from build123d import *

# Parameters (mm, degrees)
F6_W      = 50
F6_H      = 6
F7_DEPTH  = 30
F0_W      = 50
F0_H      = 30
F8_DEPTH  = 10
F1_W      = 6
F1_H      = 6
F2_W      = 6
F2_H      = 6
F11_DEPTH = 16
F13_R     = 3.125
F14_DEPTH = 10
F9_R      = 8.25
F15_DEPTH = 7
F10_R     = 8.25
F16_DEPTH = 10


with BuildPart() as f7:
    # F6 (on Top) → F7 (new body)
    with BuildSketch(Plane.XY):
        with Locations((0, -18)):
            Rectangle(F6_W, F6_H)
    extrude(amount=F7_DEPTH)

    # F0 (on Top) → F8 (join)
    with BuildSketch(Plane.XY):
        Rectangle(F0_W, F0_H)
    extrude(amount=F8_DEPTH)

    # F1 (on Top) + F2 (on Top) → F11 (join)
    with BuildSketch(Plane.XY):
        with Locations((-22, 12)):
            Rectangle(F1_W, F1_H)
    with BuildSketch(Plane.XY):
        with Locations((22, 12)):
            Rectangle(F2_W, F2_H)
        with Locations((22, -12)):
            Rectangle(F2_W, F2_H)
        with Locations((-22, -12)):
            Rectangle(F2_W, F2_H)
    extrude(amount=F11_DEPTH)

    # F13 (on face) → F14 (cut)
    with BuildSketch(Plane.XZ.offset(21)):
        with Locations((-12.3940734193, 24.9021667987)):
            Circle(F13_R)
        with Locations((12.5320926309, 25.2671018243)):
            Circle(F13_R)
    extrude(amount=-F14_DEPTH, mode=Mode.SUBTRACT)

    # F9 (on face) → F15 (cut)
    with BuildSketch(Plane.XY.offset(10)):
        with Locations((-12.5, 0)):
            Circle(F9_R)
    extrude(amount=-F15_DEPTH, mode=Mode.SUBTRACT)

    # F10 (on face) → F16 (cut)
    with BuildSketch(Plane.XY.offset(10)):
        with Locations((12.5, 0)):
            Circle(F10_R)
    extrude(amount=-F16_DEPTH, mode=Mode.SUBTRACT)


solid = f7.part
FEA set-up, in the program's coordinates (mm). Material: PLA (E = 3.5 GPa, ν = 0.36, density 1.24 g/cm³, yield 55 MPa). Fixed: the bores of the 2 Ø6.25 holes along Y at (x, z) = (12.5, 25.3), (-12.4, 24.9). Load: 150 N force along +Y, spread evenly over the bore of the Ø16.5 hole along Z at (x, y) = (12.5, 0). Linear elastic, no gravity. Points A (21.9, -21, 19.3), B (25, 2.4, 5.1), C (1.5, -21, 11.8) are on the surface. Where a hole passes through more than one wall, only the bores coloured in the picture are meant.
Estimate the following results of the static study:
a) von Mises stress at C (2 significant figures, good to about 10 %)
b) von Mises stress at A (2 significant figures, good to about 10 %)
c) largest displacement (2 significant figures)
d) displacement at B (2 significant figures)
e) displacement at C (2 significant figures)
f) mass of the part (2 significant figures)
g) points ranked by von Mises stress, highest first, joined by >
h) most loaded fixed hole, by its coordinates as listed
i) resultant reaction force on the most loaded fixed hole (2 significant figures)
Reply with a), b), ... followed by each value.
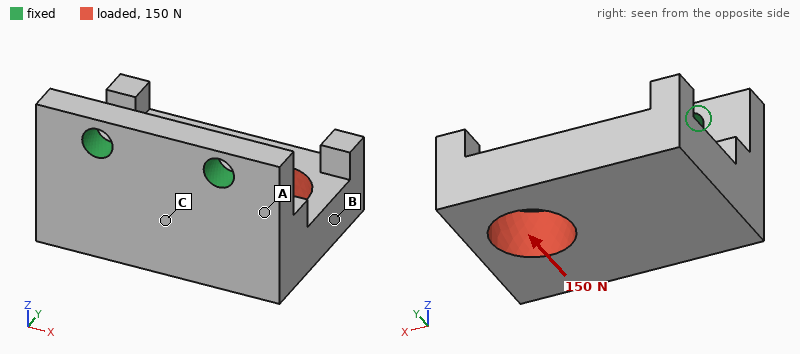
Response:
a) 3.2 MPa
b) 5.8 MPa
c) 0.38 mm
d) 0.27 mm
e) 0.072 mm
f) 26 g
g) A > C > B
h) (12.5, 25.3)
i) 130 N
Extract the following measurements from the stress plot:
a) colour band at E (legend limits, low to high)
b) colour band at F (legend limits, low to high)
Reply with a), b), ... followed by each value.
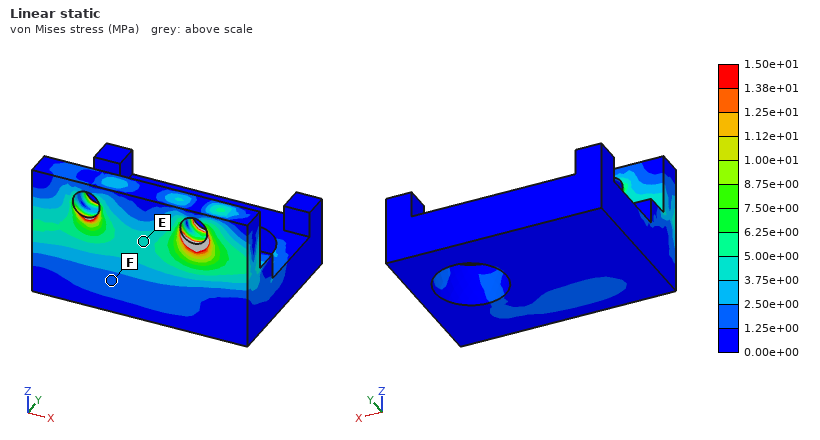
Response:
a) 3.75e+00 to 5.00e+00 MPa
b) 1.25e+00 to 2.50e+00 MPa
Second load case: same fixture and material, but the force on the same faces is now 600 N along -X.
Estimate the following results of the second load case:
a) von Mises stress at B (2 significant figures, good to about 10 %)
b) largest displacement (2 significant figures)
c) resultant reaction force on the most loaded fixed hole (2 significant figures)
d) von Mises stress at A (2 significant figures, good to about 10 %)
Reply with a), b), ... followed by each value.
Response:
a) 6.2 MPa
b) 0.62 mm
c) 580 N
d) 8.0 MPa
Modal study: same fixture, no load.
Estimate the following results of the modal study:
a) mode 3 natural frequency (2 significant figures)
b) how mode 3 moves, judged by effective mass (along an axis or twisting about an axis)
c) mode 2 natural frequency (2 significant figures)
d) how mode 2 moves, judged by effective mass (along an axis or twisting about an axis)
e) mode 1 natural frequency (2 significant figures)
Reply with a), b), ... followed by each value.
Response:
a) 2600 Hz
b) along Y
c) 1400 Hz
d) along X
e) 740 Hz
